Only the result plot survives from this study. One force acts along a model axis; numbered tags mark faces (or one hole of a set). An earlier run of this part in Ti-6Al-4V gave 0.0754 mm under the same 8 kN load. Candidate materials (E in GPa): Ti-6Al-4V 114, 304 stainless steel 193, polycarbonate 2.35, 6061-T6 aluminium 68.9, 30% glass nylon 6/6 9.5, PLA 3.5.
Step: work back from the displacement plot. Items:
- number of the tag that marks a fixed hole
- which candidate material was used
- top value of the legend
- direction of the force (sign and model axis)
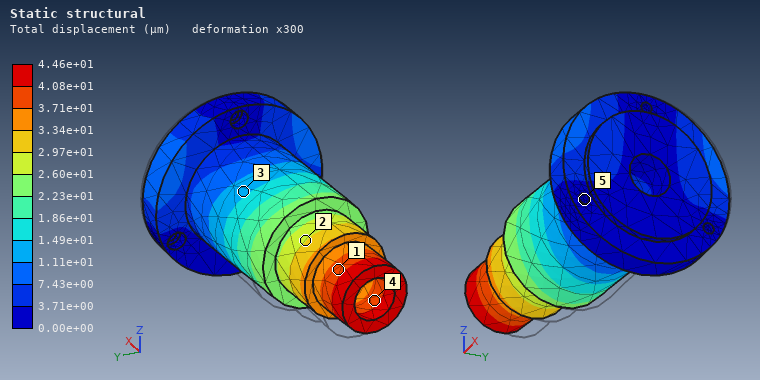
5
304 stainless steel
4.46e+01 µm
-Y
